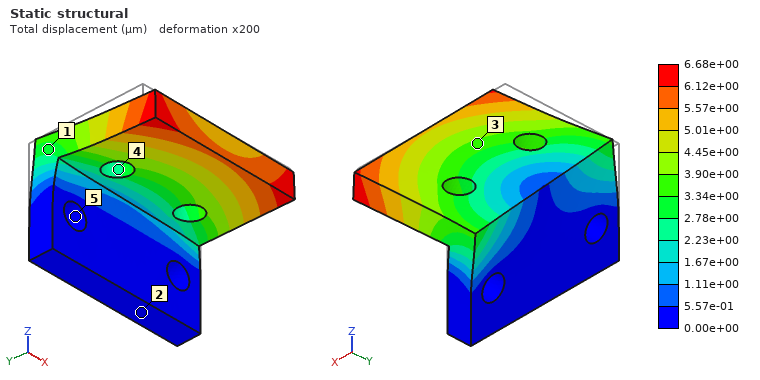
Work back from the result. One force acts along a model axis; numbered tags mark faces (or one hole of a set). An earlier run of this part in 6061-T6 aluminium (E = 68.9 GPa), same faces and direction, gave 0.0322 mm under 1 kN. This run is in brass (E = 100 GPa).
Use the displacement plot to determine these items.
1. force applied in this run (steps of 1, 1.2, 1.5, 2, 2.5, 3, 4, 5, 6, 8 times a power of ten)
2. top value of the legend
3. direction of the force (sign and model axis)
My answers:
300 N
6.68e+00 µm
+X
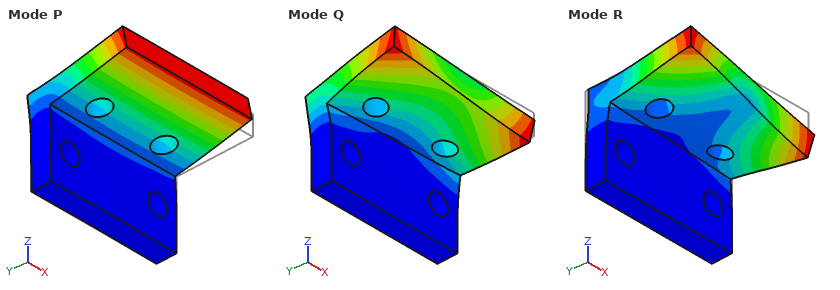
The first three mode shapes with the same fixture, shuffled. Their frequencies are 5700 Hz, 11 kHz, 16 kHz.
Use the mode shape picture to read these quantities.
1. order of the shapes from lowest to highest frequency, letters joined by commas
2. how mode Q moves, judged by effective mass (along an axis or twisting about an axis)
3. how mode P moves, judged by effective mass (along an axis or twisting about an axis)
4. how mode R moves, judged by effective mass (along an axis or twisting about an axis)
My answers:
P, Q, R
along X
along Z
along X
